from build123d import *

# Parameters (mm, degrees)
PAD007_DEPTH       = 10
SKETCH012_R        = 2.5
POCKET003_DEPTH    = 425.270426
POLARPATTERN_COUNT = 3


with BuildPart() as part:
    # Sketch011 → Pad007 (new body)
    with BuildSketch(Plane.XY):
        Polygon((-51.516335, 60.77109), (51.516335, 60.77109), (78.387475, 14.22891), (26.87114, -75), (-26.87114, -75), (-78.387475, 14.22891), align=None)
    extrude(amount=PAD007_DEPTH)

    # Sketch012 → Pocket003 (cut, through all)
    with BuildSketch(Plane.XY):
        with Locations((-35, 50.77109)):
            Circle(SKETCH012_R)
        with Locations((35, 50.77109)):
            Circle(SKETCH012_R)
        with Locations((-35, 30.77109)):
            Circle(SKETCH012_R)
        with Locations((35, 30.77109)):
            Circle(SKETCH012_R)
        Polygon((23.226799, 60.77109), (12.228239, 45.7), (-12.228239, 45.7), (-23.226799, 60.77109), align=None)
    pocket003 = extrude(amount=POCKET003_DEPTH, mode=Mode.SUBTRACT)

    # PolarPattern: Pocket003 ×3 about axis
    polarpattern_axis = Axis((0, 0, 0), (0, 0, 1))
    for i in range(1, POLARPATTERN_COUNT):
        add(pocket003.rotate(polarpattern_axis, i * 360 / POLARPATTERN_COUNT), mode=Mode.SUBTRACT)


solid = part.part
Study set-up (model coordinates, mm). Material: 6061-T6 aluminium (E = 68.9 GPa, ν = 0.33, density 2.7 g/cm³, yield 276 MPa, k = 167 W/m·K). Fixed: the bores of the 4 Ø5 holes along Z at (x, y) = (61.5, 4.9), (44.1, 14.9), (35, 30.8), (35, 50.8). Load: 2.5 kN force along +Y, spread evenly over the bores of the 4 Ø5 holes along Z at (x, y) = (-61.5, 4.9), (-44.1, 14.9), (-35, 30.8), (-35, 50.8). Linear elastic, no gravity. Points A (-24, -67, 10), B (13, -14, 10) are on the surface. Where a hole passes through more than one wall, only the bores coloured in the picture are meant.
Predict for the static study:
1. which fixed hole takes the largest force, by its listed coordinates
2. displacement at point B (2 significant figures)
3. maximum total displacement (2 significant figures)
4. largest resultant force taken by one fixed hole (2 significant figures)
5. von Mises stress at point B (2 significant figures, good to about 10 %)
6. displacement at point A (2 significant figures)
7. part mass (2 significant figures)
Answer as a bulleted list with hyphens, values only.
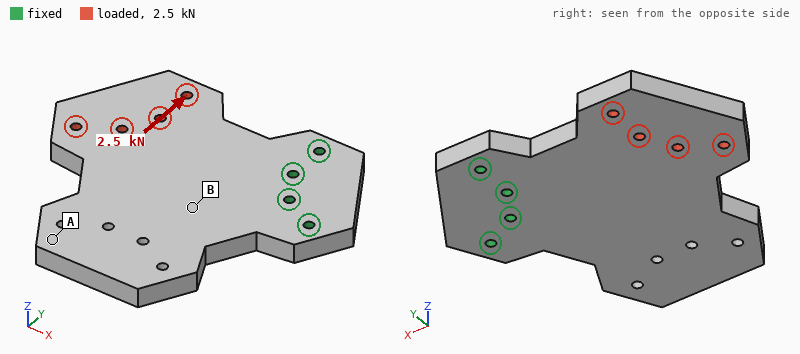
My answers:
- (35, 50.8)
- 19 µm
- 63 µm
- 3.5 kN
- 8.1 MPa
- 52 µm
- 370 g
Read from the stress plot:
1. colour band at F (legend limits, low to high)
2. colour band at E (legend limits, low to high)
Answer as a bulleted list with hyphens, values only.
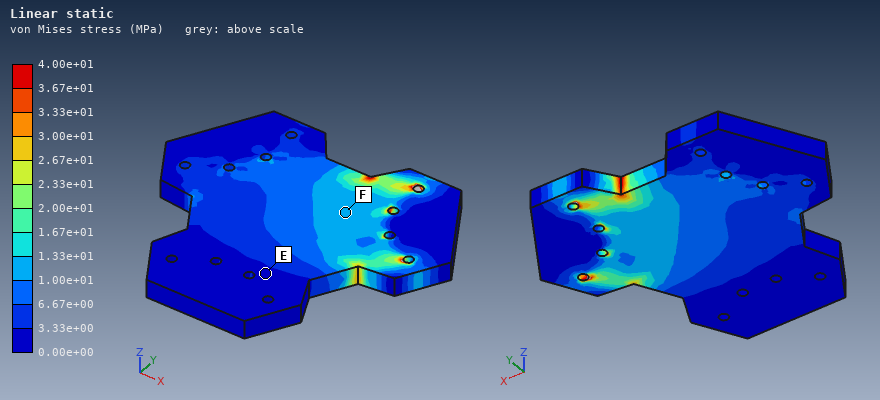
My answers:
- 1.00e+01 to 1.33e+01 MPa
- 0.00e+00 to 3.33e+00 MPa
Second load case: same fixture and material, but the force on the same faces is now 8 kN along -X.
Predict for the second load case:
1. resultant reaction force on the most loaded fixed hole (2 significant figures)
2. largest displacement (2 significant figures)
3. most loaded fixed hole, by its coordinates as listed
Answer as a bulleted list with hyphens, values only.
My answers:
- 3.0 kN
- 27 µm
- (35, 30.8)
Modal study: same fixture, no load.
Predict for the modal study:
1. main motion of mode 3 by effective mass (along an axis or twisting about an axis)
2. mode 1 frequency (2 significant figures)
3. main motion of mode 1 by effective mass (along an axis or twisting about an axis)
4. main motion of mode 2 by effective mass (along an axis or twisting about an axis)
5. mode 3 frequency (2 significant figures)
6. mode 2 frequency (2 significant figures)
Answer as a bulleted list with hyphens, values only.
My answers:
- along Y
- 600 Hz
- along Z
- twisting about X
- 2600 Hz
- 950 Hz
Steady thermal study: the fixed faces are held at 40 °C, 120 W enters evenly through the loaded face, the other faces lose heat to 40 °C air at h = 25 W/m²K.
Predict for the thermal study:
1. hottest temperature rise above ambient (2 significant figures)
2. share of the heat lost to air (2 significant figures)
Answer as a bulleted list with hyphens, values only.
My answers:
- 75 K
- 23 %
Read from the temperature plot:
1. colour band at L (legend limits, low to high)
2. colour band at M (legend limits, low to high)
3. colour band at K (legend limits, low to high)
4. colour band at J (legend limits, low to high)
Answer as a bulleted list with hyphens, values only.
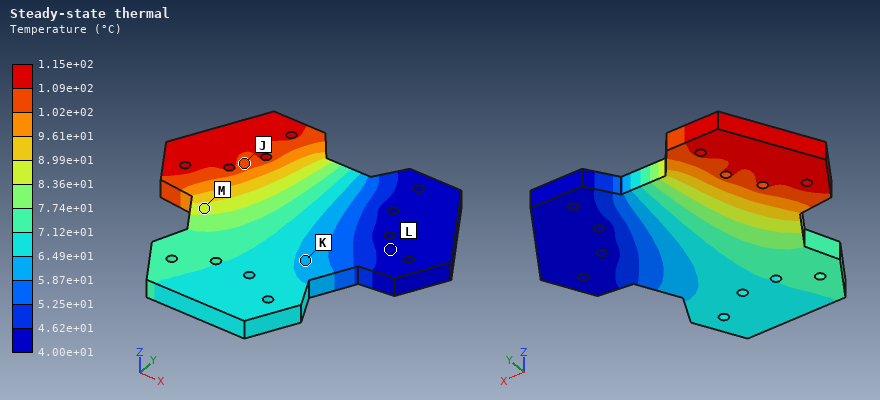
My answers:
- 4.00e+01 to 4.62e+01 °C
- 8.36e+01 to 8.99e+01 °C
- 5.87e+01 to 6.49e+01 °C
- 1.02e+02 to 1.09e+02 °C
